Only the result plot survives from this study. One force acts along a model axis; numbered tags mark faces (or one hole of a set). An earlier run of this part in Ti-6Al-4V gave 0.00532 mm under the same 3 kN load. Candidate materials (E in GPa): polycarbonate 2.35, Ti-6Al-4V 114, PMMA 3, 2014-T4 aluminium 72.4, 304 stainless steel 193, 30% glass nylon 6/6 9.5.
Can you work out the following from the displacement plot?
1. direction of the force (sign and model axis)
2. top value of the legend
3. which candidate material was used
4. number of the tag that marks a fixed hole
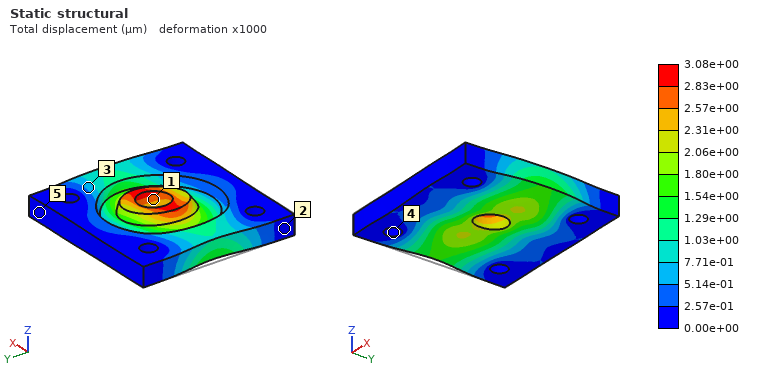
+X
3.08e+00 µm
304 stainless steel
4
